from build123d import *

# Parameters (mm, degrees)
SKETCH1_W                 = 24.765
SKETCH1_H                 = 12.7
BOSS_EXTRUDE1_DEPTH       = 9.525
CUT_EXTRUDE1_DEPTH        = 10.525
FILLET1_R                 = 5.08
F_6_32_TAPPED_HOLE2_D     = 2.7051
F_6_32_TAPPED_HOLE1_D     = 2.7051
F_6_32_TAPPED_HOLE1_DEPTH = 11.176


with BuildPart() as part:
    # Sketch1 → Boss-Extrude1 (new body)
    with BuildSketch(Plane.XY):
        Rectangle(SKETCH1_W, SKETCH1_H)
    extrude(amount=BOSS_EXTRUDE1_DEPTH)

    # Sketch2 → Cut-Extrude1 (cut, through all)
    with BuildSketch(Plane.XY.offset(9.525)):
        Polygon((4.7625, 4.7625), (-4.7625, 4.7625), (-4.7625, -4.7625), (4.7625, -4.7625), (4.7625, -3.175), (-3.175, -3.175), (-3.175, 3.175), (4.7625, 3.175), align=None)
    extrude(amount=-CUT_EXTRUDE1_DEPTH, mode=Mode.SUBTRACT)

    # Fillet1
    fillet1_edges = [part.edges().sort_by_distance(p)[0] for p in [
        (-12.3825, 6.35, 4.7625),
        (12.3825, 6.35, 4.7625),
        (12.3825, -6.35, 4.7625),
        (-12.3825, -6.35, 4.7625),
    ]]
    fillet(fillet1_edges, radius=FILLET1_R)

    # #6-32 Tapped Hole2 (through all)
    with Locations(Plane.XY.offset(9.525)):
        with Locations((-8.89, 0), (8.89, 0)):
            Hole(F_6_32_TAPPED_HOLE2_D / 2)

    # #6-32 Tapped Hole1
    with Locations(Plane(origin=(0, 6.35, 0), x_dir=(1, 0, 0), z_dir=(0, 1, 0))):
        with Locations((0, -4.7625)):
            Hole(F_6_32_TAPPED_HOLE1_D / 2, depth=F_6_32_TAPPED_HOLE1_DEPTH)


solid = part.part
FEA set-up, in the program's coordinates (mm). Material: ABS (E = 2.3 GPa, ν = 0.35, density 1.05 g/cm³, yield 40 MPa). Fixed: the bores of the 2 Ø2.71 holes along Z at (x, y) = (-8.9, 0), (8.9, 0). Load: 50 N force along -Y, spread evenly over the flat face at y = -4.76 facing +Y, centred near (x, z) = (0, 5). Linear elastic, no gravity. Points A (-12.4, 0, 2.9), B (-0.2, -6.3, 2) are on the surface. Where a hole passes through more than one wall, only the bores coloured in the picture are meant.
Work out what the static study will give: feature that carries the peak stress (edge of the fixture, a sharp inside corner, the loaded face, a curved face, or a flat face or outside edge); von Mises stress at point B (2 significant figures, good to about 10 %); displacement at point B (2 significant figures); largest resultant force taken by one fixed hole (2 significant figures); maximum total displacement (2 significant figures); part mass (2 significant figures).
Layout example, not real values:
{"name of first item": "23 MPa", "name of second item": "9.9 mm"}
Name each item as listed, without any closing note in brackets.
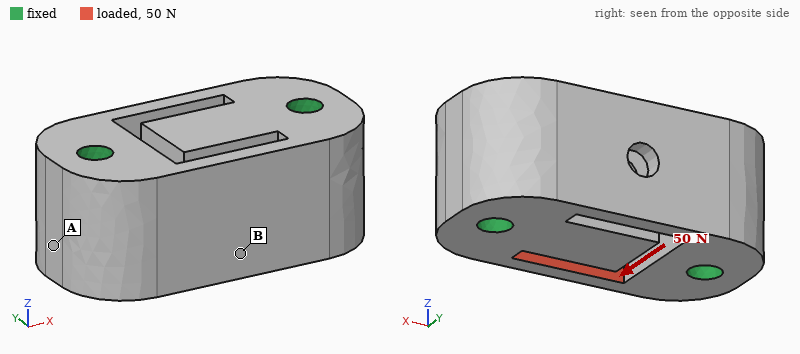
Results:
{"feature that carries the peak stress": "a flat face or outside edge", "von Mises stress at point B": "7.0 MPa", "displacement at point B": "34 µm", "largest resultant force taken by one fixed hole": "28 N", "maximum total displacement": "40 µm", "part mass": "2.4 g"}
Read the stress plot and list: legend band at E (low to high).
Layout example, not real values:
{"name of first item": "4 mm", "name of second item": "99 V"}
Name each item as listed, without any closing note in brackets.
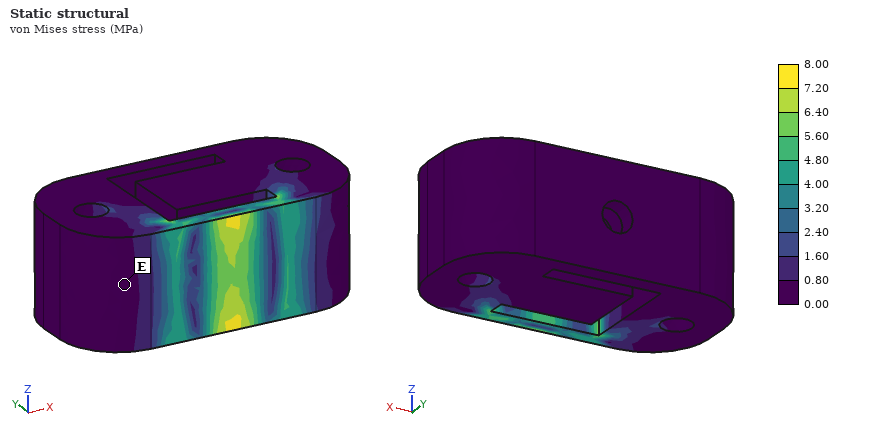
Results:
{"legend band at E": "0.00 to 0.80 MPa"}
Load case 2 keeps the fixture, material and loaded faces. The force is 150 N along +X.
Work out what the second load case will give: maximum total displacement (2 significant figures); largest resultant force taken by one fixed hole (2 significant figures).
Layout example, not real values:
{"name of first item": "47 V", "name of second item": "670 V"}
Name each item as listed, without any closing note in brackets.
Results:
{"maximum total displacement": "32 µm", "largest resultant force taken by one fixed hole": "79 N"}
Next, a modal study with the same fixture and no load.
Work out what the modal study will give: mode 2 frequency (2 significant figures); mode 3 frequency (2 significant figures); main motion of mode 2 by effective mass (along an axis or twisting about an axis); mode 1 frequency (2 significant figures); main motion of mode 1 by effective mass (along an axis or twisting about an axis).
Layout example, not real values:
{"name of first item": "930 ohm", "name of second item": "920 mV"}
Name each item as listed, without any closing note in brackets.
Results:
{"mode 2 frequency": "13 kHz", "mode 3 frequency": "17 kHz", "main motion of mode 2 by effective mass": "along Z", "mode 1 frequency": "9500 Hz", "main motion of mode 1 by effective mass": "along Y"}
